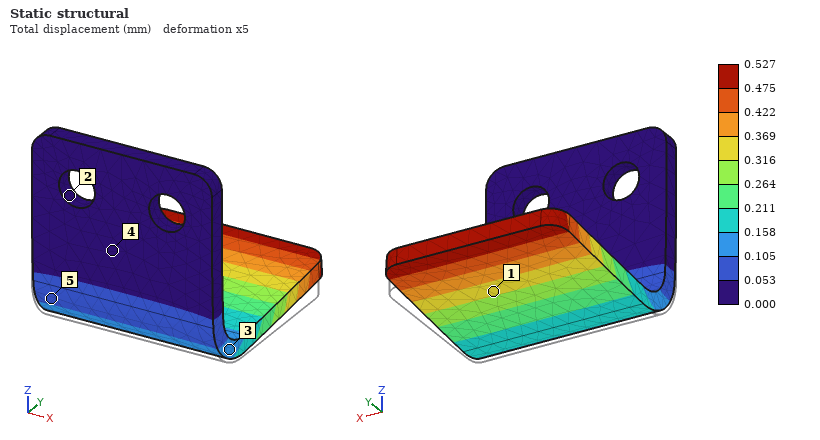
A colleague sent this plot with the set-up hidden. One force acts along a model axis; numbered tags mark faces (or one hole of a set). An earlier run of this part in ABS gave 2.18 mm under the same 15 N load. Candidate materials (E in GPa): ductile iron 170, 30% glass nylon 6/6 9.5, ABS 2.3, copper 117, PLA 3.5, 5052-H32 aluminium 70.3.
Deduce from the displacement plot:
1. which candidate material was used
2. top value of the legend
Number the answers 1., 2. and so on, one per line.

1. 30% glass nylon 6/6
2. 0.527 mm
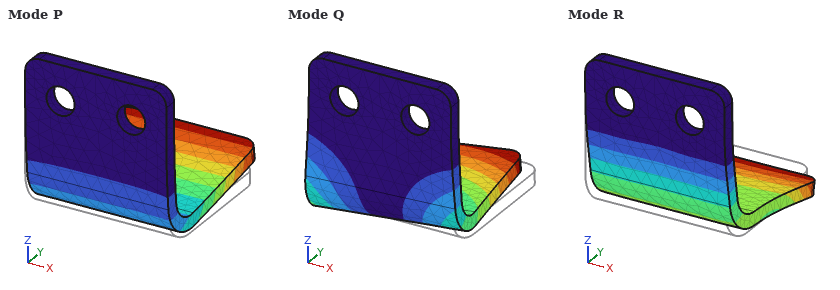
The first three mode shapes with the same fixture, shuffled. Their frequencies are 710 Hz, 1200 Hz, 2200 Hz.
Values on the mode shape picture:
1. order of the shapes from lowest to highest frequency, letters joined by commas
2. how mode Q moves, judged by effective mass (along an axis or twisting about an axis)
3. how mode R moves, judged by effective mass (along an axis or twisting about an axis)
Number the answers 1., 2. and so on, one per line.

1. P, Q, R
2. along X
3. along Y
